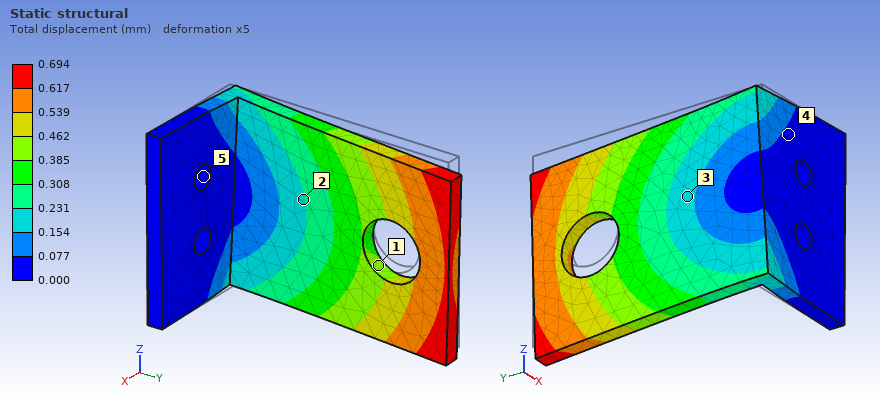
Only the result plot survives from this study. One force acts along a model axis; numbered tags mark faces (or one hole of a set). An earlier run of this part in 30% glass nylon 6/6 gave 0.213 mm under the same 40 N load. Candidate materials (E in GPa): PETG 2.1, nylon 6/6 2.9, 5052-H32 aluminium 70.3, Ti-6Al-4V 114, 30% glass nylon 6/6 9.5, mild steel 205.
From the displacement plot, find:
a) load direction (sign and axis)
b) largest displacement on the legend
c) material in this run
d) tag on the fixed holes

-Z
0.694 mm
nylon 6/6
5
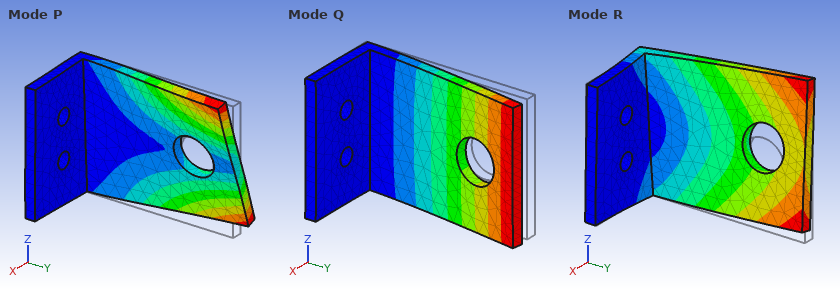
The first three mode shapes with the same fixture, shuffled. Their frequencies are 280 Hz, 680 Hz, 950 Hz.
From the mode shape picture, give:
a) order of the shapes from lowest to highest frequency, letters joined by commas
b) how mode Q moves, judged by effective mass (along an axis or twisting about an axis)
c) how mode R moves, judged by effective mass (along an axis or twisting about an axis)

Q, R, P
along X
along Z
